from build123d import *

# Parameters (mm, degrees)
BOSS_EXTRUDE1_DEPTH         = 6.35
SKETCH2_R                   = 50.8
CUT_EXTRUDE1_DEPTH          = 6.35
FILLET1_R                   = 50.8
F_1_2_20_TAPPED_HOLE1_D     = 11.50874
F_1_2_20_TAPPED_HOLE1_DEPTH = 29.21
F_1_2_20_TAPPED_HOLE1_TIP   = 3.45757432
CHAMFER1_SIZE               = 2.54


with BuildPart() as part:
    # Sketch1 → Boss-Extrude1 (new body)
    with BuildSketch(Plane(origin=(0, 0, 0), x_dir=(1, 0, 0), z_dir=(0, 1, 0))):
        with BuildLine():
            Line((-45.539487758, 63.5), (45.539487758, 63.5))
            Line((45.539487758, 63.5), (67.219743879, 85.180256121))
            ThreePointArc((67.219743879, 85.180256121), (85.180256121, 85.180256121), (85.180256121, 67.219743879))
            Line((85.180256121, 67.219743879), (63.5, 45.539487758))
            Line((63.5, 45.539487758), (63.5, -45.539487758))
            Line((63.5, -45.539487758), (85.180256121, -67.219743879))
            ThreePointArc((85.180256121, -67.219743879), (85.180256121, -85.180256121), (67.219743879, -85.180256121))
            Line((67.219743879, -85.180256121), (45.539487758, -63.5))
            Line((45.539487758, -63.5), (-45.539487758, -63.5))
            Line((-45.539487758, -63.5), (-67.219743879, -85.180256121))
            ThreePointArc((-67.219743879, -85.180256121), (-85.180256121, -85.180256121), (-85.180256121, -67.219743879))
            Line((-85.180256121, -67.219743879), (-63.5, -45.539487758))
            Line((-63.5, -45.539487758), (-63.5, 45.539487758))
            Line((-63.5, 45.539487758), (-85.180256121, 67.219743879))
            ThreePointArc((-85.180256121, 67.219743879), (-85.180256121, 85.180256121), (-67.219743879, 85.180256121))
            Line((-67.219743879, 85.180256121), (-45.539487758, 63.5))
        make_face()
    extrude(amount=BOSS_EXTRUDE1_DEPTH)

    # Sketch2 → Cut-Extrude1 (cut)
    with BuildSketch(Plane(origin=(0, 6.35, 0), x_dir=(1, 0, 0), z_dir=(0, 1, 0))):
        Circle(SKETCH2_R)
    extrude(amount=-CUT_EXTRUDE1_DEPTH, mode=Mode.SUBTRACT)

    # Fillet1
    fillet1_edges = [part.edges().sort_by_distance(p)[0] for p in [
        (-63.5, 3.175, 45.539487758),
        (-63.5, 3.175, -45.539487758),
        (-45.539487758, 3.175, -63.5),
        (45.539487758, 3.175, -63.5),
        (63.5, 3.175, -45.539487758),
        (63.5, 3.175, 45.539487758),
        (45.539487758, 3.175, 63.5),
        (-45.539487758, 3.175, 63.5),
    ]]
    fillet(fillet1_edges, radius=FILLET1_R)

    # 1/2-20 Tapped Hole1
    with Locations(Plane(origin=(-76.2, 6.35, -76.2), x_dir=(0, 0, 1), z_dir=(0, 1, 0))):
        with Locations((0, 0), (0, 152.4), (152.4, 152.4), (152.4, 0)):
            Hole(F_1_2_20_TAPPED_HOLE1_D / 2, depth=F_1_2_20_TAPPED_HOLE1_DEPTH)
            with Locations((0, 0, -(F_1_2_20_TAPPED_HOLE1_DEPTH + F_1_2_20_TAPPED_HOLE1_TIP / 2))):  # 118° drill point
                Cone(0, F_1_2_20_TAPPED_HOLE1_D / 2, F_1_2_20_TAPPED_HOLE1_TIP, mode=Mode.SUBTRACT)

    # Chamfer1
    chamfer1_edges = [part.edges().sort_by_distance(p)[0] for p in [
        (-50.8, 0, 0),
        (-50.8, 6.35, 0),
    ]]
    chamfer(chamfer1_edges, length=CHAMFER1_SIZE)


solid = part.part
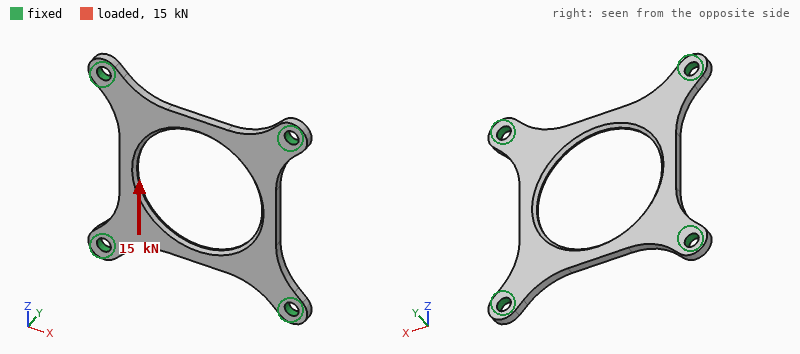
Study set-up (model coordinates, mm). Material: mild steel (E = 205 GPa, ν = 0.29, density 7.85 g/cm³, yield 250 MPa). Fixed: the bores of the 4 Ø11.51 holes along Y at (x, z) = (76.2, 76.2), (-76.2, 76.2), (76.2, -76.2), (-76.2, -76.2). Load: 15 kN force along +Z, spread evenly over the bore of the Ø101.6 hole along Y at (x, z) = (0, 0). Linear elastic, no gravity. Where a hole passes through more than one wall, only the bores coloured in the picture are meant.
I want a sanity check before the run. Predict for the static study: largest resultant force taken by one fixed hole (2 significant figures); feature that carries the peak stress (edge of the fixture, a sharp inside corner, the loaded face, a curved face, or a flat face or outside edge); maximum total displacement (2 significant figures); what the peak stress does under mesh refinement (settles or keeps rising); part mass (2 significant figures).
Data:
4.5 kN
a sharp inside corner
47 µm
keeps rising
560 g
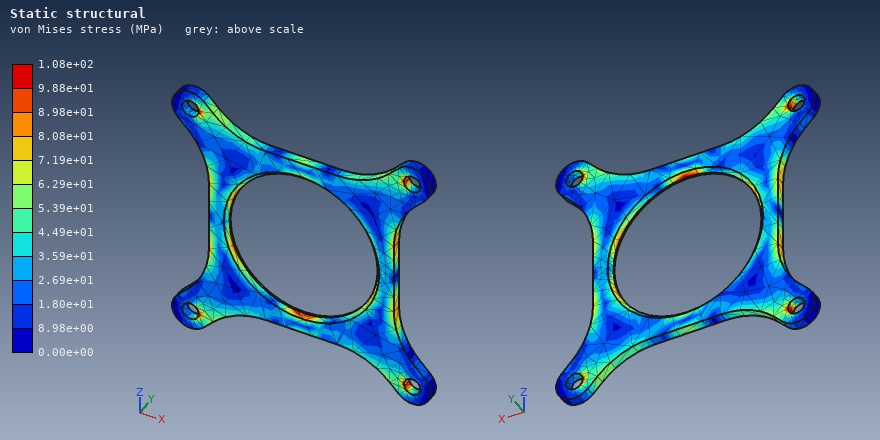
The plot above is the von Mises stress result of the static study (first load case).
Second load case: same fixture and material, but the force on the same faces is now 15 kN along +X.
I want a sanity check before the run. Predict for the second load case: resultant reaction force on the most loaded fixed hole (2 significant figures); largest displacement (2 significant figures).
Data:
4.5 kN
47 µm
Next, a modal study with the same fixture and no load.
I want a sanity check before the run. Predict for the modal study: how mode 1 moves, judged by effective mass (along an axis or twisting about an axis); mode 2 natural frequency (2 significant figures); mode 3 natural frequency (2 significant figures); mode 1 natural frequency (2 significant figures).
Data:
along Y
1700 Hz
1700 Hz
1200 Hz
